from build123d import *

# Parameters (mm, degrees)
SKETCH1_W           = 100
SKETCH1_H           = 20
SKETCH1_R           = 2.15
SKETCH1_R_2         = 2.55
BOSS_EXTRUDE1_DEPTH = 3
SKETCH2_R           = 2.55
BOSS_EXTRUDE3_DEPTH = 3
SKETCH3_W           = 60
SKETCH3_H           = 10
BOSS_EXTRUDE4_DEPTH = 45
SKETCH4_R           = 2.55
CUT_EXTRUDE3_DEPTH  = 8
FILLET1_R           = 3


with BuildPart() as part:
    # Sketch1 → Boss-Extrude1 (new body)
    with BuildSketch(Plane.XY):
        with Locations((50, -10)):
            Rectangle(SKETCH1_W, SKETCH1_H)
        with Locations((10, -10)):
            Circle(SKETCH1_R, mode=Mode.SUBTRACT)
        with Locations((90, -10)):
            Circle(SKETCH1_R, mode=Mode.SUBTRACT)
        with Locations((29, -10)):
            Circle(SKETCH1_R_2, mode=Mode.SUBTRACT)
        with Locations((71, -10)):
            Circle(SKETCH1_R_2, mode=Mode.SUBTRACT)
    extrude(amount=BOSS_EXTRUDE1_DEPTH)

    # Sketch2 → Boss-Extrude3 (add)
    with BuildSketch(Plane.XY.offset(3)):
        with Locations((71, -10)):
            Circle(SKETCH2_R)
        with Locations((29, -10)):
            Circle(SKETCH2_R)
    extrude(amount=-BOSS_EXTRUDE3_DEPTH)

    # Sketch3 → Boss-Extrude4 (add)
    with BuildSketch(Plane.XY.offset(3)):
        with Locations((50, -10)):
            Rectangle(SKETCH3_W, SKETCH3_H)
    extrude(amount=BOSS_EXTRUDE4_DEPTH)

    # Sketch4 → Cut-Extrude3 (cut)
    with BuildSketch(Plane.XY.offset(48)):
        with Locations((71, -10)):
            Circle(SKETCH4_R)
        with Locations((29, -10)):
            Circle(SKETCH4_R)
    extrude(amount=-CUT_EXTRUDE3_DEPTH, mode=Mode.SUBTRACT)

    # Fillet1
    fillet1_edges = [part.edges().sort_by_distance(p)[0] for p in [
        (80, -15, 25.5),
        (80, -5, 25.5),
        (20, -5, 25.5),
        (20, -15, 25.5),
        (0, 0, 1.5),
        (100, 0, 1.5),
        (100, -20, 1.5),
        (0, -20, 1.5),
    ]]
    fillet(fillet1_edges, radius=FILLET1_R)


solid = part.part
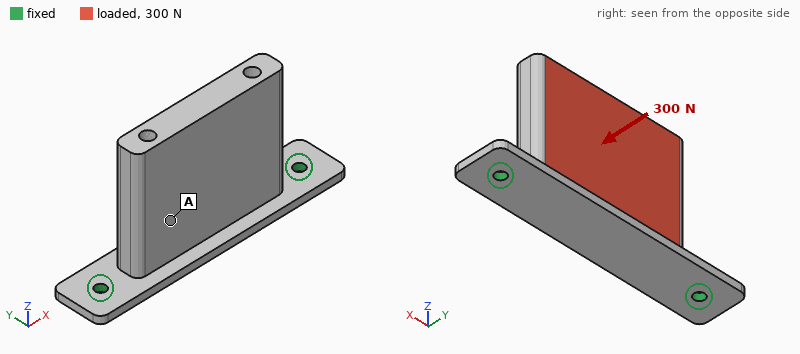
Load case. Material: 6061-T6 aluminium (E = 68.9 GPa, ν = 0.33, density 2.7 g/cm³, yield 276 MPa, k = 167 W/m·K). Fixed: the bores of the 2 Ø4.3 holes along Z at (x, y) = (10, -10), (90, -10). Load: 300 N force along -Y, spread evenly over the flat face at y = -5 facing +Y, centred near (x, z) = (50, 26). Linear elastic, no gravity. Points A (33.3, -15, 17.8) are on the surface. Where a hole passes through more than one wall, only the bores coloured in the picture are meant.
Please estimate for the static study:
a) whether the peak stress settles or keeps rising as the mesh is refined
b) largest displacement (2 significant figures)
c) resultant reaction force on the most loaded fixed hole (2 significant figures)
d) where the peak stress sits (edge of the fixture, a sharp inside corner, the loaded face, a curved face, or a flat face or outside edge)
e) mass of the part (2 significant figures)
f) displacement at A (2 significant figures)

keeps rising
0.39 mm
150 N
edge of the fixture
87 g
0.14 mm
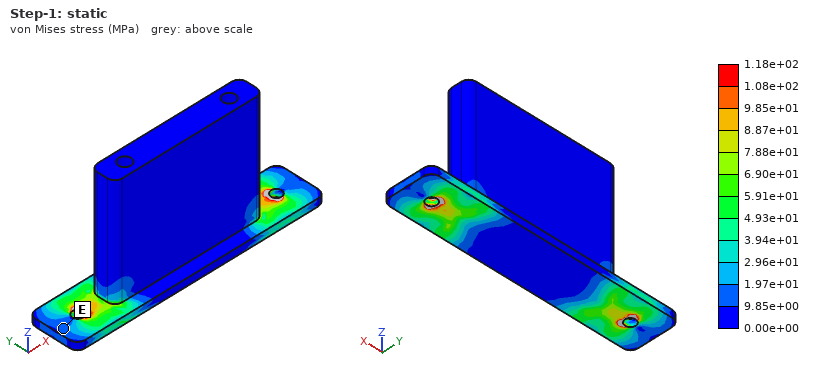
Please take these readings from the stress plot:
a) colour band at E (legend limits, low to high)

9.85e+00 to 1.97e+01 MPa
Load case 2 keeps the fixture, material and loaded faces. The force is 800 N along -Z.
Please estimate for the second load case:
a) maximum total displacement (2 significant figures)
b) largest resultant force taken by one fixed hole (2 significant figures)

0.22 mm
460 N
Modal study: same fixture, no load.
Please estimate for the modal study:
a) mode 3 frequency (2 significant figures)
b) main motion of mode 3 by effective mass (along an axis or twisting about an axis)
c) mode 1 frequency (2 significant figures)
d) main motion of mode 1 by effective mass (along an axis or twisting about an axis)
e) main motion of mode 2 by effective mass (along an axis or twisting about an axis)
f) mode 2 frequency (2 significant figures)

3500 Hz
along X
640 Hz
along Y
along Z
3100 Hz
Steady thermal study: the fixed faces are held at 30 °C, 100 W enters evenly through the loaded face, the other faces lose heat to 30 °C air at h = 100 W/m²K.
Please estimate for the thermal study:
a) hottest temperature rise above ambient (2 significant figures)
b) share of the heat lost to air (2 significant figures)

68 K
41 %
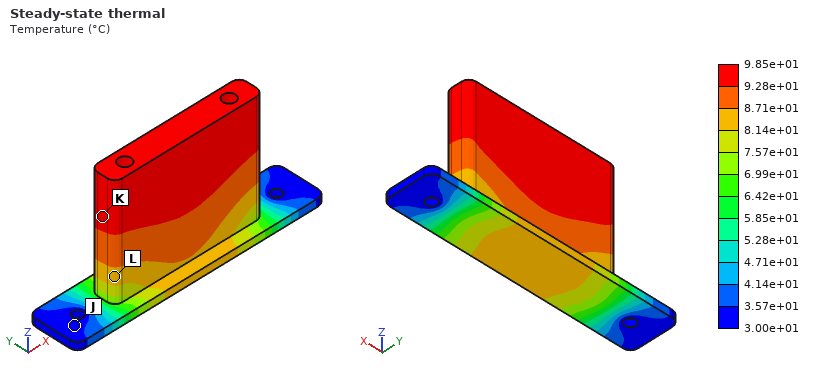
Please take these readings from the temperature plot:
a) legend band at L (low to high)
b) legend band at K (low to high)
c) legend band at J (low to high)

8.14e+01 to 8.71e+01 °C
9.28e+01 to 9.85e+01 °C
3.00e+01 to 3.57e+01 °C
